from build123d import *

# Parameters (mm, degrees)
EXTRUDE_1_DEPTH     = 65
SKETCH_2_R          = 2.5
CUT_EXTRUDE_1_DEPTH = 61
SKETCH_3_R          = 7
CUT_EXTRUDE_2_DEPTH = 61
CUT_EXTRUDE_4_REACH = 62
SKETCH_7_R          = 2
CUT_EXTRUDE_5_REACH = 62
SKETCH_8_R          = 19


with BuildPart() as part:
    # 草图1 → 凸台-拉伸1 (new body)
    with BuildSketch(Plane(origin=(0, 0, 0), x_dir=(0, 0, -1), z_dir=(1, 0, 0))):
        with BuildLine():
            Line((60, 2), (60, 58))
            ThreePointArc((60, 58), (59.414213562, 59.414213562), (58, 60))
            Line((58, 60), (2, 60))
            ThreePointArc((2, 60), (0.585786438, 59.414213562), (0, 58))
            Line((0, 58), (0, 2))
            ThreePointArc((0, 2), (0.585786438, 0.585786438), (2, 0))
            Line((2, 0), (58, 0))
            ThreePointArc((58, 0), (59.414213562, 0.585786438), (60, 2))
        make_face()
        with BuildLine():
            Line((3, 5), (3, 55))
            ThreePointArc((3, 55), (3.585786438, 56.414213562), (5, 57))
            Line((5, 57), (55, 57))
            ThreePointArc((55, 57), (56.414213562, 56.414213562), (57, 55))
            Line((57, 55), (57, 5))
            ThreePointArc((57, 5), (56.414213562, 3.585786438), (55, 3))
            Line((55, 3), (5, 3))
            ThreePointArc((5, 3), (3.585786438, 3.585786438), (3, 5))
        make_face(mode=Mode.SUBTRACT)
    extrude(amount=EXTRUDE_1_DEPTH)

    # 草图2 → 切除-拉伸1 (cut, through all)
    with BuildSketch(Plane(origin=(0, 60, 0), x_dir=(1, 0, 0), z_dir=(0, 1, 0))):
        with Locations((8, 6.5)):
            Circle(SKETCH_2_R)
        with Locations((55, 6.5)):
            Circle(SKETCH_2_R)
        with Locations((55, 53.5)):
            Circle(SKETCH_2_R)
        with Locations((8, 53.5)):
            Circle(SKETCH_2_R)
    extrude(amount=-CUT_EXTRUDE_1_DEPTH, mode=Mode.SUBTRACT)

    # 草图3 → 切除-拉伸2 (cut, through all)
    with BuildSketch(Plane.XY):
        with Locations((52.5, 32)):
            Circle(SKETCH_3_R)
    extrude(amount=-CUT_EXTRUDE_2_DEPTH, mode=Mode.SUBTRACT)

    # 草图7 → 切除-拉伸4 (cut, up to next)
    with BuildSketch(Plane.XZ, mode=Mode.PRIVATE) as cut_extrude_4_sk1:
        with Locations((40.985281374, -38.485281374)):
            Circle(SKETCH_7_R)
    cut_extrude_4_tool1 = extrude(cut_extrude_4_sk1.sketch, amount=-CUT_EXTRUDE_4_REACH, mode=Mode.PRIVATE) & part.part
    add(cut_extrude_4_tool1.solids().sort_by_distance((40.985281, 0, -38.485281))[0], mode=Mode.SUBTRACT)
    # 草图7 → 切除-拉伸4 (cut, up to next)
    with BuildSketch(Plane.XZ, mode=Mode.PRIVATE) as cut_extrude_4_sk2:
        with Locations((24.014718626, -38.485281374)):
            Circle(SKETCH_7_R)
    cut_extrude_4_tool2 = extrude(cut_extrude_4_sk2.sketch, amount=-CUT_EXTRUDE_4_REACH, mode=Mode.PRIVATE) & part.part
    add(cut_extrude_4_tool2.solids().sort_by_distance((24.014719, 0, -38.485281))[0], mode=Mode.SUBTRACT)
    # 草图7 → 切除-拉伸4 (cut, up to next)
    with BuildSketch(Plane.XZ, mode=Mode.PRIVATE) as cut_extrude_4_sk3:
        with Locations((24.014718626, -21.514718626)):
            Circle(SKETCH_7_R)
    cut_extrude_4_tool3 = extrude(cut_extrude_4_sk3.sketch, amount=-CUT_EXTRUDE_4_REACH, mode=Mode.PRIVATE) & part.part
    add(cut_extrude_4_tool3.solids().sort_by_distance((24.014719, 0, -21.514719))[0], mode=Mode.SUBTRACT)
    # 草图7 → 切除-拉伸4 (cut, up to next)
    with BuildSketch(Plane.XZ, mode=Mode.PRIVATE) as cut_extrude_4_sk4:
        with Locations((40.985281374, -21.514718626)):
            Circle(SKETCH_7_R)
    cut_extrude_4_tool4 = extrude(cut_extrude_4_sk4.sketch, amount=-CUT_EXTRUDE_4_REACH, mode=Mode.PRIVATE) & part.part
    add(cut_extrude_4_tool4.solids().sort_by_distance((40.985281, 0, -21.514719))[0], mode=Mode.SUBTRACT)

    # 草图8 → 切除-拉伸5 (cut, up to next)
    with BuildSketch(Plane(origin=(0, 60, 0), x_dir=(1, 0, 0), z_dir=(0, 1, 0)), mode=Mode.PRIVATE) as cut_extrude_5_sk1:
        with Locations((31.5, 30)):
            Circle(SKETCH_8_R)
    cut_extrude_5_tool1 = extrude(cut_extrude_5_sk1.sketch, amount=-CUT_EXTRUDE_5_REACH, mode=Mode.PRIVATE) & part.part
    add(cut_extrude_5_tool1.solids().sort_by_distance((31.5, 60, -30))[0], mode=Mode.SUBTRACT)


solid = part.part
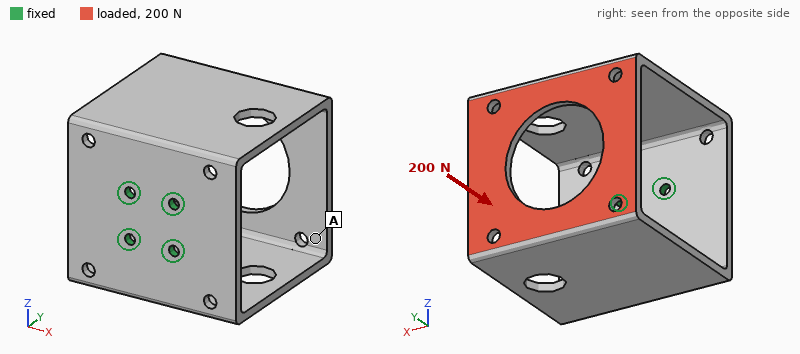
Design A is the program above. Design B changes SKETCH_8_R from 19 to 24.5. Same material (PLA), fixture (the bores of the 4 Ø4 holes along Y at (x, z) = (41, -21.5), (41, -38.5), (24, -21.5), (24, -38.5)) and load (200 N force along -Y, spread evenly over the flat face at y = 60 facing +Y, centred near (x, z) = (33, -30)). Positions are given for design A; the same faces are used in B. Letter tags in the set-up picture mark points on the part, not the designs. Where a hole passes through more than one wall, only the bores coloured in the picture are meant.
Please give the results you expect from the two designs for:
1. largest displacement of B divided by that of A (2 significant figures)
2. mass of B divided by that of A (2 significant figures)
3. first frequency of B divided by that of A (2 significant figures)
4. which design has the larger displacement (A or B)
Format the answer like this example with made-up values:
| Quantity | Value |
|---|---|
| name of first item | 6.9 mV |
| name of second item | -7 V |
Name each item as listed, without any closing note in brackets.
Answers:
| Quantity | Value |
|---|---|
| largest displacement of B divided by that of A | 1.2 |
| mass of B divided by that of A | 0.94 |
| first frequency of B divided by that of A | 1.0 |
| which design has the larger displacement | B |
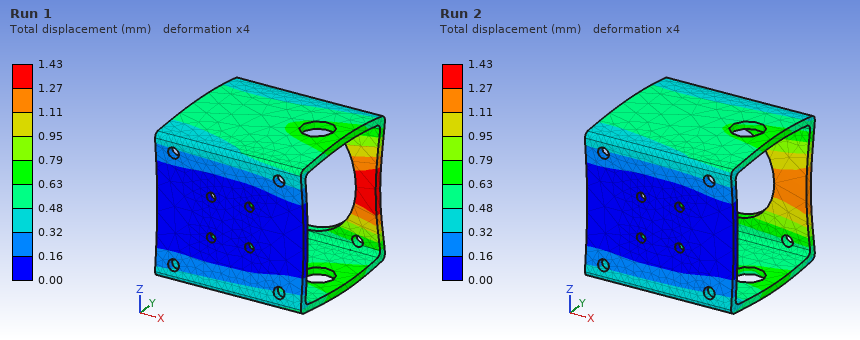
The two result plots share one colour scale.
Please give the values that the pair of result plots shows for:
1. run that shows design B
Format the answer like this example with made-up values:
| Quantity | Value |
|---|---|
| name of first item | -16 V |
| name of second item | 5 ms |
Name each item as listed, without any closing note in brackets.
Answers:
| Quantity | Value |
|---|---|
| run that shows design B | Run 1 |
